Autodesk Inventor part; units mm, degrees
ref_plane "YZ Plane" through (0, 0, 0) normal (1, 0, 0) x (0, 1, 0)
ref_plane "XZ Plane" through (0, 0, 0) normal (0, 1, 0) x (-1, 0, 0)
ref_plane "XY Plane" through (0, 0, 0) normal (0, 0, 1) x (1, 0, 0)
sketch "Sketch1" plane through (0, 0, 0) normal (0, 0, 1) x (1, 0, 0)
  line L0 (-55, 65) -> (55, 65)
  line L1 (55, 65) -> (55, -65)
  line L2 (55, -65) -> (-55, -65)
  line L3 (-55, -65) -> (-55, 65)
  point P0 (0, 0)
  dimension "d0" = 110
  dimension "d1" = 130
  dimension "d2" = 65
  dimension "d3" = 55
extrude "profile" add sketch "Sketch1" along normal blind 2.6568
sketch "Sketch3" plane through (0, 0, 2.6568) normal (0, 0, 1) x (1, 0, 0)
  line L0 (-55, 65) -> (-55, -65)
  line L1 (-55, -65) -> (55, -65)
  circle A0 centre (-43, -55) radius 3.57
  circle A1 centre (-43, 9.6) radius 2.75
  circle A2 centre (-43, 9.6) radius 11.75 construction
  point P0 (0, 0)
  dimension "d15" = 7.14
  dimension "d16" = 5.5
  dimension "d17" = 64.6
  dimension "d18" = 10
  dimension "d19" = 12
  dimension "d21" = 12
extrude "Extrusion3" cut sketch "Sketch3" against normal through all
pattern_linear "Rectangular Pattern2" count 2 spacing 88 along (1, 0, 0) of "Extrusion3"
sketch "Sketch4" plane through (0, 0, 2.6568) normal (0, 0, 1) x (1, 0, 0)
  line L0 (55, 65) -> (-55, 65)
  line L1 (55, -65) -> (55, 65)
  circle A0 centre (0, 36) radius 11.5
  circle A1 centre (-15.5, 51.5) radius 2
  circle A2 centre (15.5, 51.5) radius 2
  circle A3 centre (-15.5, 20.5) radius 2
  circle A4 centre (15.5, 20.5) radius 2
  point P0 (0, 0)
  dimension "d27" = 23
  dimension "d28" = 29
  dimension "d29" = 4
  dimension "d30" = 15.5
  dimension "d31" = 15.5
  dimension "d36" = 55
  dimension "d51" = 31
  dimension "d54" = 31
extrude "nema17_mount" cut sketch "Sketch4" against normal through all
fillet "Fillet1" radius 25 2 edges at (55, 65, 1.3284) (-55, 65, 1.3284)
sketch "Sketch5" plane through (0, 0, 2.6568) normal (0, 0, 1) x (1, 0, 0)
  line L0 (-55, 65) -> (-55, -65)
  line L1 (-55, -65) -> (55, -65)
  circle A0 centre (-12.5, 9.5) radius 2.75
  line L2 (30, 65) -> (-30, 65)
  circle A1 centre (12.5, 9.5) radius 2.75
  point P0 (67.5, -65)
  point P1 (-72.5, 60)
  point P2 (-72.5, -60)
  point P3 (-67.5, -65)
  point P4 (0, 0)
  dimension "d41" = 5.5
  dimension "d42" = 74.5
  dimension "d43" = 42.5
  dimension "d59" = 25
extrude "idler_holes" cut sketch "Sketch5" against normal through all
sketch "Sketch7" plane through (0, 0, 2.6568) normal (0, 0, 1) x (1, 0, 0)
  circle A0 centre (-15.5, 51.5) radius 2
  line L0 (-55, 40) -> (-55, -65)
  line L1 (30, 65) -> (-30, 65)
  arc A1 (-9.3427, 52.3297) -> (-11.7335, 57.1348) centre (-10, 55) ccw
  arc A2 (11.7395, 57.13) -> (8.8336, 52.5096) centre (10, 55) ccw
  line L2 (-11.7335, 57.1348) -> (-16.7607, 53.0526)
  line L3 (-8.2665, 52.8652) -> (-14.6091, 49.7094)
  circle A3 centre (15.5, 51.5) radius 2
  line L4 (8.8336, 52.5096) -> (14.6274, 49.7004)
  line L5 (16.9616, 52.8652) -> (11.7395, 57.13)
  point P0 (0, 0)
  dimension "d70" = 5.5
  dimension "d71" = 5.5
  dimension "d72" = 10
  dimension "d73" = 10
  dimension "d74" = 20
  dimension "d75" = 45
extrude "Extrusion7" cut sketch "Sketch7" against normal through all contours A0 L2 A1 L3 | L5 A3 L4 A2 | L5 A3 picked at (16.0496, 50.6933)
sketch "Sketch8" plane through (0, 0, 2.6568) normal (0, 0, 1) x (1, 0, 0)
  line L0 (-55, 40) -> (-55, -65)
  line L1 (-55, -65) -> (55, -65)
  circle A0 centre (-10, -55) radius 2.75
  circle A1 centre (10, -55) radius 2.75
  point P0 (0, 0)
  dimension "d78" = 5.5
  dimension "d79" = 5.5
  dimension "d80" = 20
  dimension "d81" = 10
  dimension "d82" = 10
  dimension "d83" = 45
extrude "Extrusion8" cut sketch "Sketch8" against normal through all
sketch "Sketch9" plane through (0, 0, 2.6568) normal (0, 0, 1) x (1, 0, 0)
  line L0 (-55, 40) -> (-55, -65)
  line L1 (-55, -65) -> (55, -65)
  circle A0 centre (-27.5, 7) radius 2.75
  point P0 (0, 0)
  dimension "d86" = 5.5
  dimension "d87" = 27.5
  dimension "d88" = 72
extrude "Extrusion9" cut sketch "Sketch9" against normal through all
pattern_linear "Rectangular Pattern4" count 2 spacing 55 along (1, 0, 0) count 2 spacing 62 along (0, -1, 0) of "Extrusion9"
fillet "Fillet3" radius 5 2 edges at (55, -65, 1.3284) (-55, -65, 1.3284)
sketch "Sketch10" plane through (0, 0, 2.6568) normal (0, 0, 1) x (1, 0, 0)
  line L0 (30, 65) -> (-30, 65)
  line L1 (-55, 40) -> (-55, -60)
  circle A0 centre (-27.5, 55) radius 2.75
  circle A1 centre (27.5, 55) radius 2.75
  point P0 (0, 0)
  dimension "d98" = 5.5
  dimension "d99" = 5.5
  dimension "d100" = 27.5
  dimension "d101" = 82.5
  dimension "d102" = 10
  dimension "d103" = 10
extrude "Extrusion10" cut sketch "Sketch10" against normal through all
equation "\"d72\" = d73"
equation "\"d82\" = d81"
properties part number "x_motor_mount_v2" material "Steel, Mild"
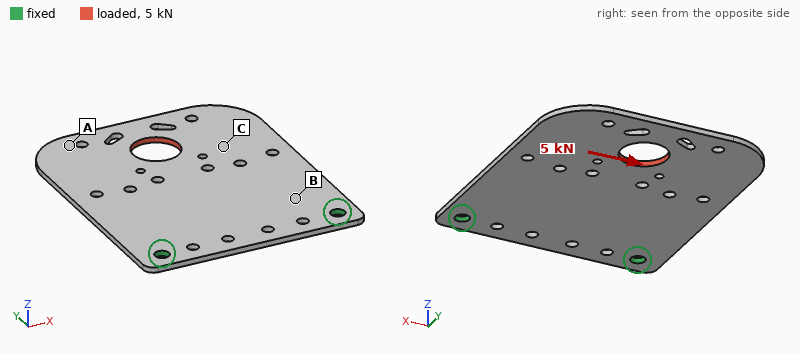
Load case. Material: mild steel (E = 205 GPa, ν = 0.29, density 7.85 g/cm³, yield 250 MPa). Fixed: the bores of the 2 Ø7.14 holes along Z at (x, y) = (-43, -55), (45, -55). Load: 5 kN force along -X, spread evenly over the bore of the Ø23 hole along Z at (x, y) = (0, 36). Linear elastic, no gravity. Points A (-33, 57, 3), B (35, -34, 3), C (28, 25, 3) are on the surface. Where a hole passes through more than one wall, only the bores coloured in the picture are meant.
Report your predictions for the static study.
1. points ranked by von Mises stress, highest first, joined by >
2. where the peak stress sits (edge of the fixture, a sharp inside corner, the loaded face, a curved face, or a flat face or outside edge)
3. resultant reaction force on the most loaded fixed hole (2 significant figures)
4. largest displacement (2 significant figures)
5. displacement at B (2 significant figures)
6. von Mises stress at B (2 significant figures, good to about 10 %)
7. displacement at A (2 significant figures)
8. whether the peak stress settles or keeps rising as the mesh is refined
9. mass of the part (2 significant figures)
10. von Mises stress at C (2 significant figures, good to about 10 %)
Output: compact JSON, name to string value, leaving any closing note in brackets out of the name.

{"points ranked by von Mises stress, highest first, joined by >": "B > C > A", "where the peak stress sits": "edge of the fixture", "resultant reaction force on the most loaded fixed hole": "5.6 kN", "largest displacement": "66 µm", "displacement at B": "10 µm", "von Mises stress at B": "56 MPa", "displacement at A": "62 µm", "whether the peak stress settles or keeps rising as the mesh is refined": "keeps rising", "mass of the part": "270 g", "von Mises stress at C": "32 MPa"}
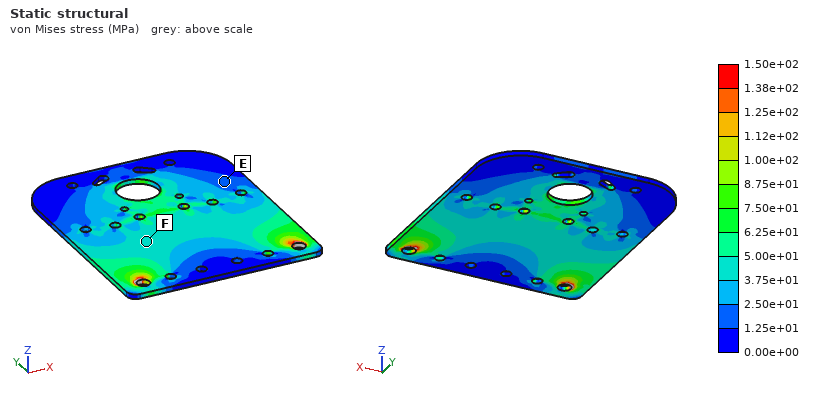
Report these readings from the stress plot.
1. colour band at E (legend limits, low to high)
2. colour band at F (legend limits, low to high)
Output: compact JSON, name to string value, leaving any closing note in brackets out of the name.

{"colour band at E": "1.25e+01 to 2.50e+01 MPa", "colour band at F": "3.75e+01 to 5.00e+01 MPa"}
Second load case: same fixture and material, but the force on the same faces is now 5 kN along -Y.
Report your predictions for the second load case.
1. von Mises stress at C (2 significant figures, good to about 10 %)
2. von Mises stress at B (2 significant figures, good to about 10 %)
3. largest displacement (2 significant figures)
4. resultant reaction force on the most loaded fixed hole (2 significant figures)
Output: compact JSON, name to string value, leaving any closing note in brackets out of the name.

{"von Mises stress at C": "21 MPa", "von Mises stress at B": "27 MPa", "largest displacement": "19 µm", "resultant reaction force on the most loaded fixed hole": "2.6 kN"}
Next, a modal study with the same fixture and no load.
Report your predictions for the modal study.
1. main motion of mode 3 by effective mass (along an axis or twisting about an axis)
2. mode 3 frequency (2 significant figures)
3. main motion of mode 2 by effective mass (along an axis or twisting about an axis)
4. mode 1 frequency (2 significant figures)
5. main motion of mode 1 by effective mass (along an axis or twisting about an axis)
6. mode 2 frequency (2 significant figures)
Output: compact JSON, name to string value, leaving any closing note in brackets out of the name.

{"main motion of mode 3 by effective mass": "along Z", "mode 3 frequency": "890 Hz", "main motion of mode 2 by effective mass": "twisting about Y", "mode 1 frequency": "150 Hz", "main motion of mode 1 by effective mass": "along Z", "mode 2 frequency": "430 Hz"}
